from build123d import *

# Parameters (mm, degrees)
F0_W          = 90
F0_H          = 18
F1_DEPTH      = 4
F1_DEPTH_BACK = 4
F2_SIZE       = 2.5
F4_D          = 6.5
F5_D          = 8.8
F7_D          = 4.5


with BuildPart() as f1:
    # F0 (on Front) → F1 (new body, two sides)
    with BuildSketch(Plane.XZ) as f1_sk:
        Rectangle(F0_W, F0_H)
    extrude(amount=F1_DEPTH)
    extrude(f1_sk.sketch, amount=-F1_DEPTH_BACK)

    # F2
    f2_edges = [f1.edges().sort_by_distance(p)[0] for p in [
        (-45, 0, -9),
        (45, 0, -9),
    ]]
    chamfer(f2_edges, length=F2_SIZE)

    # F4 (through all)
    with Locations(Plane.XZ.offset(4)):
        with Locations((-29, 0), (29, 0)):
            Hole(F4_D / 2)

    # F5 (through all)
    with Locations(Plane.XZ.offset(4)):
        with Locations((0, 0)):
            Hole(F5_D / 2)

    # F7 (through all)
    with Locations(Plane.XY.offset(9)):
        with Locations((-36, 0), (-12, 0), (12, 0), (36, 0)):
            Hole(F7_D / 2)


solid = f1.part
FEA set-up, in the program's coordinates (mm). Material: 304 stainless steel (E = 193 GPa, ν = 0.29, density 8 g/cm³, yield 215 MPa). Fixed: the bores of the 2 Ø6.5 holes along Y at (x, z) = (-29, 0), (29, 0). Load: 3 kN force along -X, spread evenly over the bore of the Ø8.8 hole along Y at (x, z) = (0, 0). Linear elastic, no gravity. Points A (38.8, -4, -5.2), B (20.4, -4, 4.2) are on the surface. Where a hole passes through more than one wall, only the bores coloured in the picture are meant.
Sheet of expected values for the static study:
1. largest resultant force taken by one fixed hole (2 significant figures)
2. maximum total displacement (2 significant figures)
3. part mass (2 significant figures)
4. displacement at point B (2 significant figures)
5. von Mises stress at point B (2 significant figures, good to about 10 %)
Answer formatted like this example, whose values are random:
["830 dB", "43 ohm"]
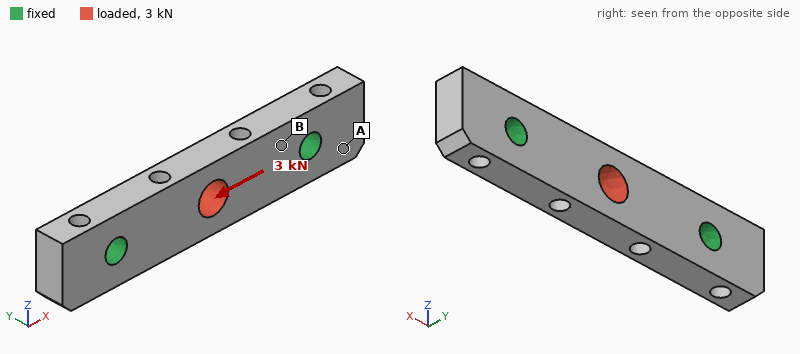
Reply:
["1.5 kN", "2.1 µm", "86 g", "0.50 µm", "12 MPa"]
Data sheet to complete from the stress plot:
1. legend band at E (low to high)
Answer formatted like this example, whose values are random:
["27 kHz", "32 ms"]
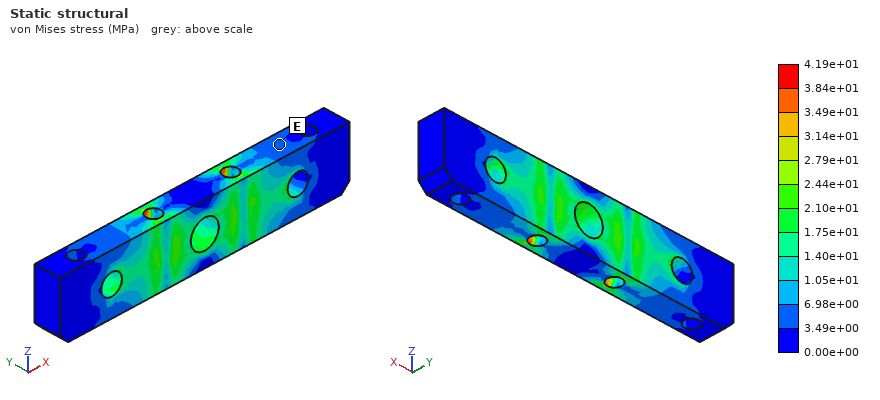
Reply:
["3.49e+00 to 6.98e+00 MPa"]
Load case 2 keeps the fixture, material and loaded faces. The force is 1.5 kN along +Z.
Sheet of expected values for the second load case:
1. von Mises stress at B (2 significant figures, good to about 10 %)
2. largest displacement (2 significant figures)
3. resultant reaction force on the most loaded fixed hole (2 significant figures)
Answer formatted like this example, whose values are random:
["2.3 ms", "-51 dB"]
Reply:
["11 MPa", "5.7 µm", "750 N"]
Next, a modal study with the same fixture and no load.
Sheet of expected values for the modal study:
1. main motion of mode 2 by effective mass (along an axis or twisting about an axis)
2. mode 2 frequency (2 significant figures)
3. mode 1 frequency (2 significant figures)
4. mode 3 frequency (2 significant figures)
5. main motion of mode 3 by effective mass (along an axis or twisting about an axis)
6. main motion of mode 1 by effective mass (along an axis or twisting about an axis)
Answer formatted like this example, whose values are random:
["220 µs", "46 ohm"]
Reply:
["along Z", "17 kHz", "11 kHz", "20 kHz", "twisting about X", "along Y"]
